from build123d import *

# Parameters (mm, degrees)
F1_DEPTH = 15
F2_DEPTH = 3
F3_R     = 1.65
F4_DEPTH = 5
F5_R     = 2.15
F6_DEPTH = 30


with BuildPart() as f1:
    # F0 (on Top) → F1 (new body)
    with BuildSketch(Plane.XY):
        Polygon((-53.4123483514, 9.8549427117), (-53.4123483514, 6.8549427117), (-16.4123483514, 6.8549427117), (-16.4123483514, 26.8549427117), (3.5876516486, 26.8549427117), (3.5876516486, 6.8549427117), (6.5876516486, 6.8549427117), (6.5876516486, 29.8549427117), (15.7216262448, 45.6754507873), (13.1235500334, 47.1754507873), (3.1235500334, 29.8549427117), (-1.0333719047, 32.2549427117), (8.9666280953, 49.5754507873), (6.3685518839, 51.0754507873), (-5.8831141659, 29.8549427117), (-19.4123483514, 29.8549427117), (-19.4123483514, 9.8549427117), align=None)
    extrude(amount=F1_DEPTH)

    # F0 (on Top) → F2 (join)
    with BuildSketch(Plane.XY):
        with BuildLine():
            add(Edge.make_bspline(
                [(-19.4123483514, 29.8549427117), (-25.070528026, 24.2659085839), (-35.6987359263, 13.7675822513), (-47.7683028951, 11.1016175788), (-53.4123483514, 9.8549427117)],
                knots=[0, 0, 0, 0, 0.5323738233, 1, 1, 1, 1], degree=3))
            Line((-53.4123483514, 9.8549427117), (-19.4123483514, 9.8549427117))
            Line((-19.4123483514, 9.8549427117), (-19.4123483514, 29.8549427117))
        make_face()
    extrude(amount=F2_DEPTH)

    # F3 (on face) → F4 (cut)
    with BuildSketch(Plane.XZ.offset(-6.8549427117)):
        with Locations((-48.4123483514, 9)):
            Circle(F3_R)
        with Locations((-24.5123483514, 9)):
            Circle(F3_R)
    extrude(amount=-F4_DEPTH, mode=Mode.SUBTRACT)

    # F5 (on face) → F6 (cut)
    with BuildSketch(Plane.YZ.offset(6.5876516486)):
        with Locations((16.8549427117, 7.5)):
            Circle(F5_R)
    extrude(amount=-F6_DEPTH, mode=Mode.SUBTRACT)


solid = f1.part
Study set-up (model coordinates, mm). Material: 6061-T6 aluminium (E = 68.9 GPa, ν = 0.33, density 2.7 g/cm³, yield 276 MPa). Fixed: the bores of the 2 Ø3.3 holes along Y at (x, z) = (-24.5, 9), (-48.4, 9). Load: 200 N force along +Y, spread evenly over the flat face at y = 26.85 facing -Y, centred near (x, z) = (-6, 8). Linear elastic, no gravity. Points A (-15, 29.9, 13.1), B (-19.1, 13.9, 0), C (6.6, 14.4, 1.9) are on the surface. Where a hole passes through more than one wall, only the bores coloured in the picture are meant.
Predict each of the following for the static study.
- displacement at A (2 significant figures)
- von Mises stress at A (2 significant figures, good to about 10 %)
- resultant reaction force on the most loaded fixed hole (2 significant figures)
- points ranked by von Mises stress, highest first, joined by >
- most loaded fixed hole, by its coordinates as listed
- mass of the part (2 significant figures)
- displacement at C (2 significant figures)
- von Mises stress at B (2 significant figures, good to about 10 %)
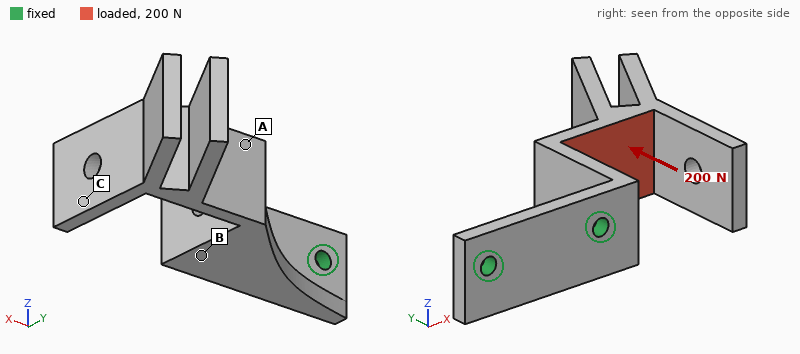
0.085 mm
58 MPa
320 N
A > B > C
(-24.5, 9)
19 g
0.30 mm
22 MPa
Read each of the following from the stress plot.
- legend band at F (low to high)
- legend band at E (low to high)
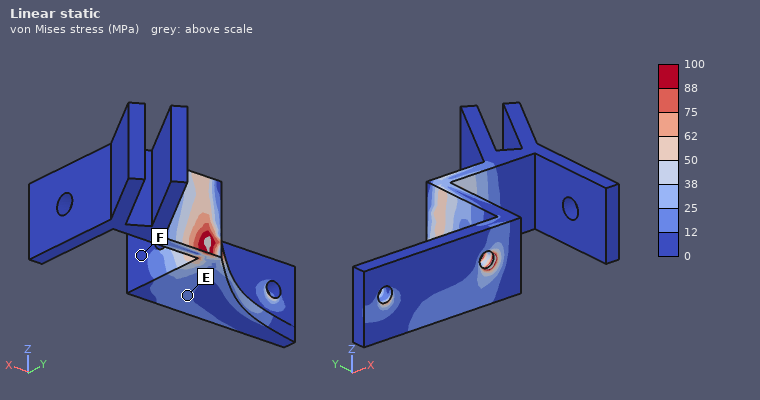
0 to 12 MPa
12 to 25 MPa
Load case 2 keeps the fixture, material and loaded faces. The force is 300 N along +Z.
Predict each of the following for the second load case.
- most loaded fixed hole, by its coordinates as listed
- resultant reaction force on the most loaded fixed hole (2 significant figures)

(-24.5, 9)
480 N
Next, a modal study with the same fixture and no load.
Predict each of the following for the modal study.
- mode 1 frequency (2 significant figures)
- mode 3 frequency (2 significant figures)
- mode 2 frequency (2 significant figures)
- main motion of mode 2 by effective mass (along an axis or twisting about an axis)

780 Hz
2200 Hz
1200 Hz
along Z
